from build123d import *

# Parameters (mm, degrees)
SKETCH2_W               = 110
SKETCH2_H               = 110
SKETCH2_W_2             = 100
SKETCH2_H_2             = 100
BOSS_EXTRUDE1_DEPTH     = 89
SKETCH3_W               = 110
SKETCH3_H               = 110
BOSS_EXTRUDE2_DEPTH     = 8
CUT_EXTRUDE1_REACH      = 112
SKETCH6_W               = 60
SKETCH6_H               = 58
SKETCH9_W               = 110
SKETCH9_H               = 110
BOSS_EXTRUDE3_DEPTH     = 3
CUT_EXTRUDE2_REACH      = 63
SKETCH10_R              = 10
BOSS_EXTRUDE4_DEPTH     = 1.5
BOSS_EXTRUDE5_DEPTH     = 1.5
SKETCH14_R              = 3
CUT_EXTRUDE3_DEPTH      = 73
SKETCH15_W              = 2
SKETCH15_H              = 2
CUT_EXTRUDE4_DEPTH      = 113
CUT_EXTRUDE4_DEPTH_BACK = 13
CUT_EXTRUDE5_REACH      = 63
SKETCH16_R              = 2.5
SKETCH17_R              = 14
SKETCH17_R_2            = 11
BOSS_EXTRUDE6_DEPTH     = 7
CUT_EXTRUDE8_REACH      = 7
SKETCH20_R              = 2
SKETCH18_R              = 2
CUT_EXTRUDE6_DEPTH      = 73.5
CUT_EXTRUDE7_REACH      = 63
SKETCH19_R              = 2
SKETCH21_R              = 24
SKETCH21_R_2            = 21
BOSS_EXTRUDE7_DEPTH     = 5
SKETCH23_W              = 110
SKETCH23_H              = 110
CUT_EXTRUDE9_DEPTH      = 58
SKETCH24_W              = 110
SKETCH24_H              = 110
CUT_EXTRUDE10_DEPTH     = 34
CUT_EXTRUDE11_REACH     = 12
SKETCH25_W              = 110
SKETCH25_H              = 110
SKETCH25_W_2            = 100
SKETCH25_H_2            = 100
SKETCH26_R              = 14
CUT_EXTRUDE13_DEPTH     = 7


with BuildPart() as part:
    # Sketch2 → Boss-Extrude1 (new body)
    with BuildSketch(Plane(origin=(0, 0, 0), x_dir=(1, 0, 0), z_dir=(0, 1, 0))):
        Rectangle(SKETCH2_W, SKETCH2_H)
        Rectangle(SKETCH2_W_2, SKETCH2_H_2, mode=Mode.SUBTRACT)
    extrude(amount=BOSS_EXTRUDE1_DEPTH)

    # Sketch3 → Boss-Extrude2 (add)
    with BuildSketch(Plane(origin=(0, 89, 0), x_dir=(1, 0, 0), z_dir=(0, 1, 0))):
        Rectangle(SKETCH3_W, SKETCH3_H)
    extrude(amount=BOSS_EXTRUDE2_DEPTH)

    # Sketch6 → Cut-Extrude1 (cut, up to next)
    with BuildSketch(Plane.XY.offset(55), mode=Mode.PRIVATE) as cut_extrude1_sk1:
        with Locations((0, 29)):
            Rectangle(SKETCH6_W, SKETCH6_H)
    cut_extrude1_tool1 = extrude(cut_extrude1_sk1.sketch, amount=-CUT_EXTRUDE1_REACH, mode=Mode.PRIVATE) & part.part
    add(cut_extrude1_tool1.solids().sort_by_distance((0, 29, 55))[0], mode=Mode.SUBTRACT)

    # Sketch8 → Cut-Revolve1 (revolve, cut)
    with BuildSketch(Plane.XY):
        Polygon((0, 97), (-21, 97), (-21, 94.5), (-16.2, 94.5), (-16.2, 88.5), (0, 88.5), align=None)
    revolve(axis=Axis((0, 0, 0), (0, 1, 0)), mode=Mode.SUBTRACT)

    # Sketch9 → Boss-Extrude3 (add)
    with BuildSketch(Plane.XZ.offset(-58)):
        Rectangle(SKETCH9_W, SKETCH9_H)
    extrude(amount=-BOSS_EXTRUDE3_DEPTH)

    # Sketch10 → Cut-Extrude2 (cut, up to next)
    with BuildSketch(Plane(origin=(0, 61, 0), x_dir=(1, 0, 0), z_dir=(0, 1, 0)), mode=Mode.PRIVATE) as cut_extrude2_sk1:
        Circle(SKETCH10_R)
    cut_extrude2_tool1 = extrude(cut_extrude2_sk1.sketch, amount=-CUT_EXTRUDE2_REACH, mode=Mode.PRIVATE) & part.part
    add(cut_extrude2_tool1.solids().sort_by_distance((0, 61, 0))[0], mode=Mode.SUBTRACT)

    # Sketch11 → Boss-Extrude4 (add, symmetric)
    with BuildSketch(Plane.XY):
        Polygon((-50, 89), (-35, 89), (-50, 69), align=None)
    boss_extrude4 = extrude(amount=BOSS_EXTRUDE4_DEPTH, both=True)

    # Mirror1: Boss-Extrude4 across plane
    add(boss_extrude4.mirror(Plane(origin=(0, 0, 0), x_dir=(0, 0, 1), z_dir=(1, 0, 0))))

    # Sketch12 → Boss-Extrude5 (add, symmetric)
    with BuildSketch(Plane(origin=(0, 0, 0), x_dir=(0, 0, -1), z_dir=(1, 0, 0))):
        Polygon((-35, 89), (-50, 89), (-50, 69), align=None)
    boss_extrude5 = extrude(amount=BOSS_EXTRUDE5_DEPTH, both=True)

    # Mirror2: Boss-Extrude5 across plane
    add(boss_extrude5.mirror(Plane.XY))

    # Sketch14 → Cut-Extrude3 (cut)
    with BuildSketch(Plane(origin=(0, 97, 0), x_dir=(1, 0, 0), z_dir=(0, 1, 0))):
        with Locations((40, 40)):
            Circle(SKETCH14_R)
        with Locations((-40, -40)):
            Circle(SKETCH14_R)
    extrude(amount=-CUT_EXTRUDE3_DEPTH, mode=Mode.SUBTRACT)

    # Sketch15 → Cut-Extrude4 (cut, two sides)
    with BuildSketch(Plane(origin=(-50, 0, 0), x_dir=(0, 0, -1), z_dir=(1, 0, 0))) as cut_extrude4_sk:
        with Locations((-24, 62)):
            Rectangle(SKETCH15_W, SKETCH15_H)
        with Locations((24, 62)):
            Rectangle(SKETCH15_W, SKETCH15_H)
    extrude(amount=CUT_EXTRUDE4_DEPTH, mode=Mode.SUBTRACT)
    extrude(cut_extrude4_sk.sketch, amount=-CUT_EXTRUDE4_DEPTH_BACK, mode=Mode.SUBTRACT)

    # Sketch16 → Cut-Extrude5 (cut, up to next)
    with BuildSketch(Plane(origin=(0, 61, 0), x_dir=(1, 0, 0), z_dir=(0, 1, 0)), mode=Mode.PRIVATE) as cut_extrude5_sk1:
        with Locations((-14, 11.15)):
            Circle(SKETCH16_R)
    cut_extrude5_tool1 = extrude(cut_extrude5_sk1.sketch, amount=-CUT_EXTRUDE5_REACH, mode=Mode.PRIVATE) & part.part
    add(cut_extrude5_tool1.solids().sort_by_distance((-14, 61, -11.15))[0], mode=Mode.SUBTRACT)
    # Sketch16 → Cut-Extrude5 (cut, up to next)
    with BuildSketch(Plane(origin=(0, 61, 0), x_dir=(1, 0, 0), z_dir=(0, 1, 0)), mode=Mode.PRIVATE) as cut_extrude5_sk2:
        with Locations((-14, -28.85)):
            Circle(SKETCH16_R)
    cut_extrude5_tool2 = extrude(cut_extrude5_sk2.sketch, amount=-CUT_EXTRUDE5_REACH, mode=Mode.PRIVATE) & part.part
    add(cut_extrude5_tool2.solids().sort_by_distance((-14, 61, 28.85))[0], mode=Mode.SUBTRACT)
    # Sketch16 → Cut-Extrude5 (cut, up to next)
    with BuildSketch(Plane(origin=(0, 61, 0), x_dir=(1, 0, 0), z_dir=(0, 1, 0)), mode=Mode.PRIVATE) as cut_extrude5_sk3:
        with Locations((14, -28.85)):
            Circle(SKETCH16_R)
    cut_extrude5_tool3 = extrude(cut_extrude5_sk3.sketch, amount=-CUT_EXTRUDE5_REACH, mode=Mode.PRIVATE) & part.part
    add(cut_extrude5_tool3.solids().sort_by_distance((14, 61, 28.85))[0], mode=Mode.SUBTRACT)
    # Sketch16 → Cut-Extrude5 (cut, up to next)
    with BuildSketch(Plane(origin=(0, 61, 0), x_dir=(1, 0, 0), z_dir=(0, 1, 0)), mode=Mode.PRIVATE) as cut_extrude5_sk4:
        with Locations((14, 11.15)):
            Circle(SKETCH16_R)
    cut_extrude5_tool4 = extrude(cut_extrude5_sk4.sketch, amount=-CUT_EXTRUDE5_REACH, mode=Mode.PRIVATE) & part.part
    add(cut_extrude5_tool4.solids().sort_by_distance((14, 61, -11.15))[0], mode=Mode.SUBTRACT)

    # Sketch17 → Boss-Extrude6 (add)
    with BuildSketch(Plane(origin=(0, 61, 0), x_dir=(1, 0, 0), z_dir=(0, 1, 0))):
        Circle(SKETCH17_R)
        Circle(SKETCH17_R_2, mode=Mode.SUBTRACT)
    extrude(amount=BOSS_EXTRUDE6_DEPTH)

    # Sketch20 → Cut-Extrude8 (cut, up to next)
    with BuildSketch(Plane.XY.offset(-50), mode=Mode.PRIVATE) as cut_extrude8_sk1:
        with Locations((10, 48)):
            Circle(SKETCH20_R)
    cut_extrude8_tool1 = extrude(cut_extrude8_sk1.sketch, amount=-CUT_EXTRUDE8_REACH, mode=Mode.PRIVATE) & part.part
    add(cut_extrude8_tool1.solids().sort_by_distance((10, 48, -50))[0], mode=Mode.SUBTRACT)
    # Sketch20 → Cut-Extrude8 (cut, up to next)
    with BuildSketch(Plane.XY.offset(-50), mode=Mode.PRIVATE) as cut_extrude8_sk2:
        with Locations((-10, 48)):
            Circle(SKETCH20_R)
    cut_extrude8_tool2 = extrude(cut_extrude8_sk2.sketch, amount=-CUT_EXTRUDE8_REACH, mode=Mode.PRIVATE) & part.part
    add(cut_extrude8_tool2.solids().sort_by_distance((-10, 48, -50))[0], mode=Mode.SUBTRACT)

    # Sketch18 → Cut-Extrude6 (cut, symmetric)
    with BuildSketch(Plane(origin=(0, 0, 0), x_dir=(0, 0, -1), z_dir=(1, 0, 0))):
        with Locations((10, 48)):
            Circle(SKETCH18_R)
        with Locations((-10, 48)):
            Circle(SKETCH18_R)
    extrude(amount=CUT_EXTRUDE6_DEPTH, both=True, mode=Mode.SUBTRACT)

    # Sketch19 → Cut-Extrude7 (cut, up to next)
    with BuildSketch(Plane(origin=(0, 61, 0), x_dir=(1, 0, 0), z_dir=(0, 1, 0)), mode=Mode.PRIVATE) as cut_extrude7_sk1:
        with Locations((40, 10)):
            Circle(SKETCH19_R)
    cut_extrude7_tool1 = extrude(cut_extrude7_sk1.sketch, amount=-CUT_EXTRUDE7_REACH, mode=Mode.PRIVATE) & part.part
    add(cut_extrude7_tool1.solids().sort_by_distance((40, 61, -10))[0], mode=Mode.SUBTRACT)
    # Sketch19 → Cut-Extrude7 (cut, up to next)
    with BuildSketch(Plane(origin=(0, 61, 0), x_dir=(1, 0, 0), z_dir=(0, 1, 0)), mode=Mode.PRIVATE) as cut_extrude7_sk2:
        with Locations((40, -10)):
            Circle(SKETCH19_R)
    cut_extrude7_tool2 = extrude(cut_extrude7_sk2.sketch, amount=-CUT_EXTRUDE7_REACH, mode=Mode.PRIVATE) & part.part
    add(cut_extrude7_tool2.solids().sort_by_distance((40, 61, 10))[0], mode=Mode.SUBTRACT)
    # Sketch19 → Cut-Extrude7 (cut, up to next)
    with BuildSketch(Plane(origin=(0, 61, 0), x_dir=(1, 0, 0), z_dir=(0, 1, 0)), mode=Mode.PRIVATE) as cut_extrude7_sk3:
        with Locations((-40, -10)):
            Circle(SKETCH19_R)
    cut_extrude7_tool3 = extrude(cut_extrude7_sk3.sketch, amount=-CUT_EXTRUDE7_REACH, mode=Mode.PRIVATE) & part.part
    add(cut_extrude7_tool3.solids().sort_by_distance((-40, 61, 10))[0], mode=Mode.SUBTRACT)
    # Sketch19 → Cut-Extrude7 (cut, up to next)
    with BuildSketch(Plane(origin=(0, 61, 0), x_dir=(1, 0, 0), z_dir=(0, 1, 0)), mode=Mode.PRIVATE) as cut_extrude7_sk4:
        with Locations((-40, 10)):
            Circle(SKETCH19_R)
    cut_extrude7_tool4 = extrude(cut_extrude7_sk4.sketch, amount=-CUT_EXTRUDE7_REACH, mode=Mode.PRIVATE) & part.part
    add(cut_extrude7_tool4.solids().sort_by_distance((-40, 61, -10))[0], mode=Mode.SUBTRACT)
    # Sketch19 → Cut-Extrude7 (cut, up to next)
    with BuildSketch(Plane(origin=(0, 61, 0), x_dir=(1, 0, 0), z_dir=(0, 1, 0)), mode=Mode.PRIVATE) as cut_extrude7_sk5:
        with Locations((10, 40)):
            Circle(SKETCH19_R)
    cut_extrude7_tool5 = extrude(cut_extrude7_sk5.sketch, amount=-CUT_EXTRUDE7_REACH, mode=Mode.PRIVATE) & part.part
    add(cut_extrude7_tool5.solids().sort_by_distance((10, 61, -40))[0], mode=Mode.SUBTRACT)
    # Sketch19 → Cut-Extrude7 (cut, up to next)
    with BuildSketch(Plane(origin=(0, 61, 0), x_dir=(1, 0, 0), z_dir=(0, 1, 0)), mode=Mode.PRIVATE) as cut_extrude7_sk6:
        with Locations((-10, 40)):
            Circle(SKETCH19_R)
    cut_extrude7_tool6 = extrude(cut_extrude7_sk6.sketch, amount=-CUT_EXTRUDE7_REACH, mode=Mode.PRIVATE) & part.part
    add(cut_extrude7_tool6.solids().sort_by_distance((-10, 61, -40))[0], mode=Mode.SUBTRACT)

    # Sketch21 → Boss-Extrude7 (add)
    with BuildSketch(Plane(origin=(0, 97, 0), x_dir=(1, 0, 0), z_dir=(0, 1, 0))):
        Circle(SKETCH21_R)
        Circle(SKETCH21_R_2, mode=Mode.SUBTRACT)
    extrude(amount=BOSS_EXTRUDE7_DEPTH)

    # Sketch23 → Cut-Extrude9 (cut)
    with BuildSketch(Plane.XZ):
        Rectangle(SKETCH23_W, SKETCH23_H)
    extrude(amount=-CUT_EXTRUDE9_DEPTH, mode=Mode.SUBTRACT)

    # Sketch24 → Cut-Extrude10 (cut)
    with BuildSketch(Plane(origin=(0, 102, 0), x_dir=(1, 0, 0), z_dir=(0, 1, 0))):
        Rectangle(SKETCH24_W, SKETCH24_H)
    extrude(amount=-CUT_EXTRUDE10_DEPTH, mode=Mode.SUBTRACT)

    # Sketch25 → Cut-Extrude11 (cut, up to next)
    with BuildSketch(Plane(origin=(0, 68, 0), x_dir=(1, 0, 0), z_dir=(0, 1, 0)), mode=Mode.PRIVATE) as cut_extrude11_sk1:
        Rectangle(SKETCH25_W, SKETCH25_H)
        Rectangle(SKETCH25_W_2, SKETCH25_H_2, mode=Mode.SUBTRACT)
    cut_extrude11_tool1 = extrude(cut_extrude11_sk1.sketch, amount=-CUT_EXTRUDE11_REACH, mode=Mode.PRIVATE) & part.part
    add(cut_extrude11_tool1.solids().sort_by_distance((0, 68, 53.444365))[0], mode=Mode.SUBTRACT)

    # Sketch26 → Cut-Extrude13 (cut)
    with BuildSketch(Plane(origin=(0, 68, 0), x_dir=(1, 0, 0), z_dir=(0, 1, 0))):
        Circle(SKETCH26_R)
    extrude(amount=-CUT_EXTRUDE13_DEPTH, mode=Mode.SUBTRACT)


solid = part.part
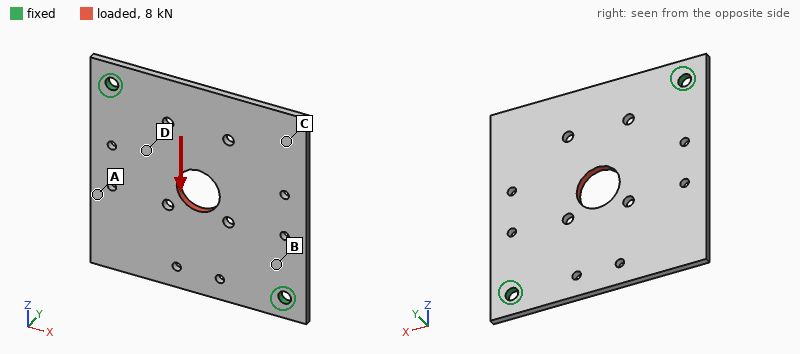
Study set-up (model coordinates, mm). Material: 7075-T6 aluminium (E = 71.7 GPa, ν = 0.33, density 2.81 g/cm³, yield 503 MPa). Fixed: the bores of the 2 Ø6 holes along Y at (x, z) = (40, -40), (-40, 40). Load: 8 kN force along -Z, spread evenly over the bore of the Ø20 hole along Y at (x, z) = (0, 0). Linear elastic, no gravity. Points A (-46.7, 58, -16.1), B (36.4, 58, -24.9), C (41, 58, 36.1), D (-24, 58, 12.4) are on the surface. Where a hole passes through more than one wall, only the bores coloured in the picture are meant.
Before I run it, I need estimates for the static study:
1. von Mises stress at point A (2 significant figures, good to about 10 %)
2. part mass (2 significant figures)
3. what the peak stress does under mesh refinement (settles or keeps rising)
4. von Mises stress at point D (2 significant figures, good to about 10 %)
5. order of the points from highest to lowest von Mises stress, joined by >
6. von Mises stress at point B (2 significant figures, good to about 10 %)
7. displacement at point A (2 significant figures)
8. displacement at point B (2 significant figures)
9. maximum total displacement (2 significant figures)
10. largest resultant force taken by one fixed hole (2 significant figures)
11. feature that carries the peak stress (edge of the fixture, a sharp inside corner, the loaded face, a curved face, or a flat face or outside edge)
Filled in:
21 MPa
80 g
keeps rising
34 MPa
B > D > A > C
53 MPa
33 µm
18 µm
54 µm
4.0 kN
edge of the fixture
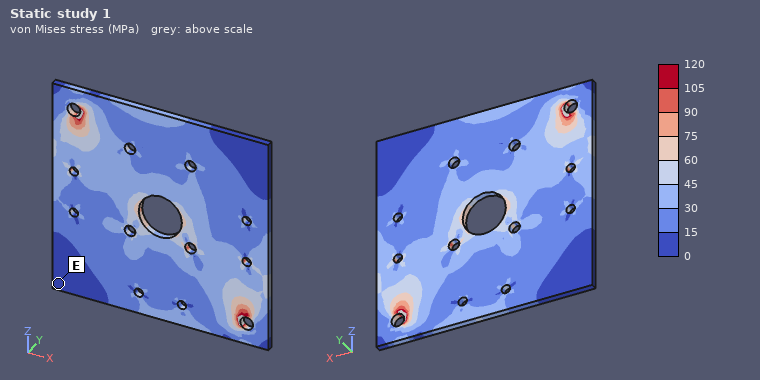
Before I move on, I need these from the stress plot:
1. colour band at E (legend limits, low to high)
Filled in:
0 to 15 MPa
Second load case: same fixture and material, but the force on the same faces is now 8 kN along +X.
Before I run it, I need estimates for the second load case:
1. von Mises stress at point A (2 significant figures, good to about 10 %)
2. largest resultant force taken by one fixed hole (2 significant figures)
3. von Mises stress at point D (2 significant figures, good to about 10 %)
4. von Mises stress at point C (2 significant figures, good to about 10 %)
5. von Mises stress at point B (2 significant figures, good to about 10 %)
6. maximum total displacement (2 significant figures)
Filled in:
24 MPa
4.0 kN
27 MPa
9.9 MPa
31 MPa
55 µm
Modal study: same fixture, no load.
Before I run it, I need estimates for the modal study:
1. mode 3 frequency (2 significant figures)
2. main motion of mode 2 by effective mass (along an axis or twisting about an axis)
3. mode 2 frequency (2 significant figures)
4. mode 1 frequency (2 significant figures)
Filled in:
1700 Hz
along Y
660 Hz
490 Hz
